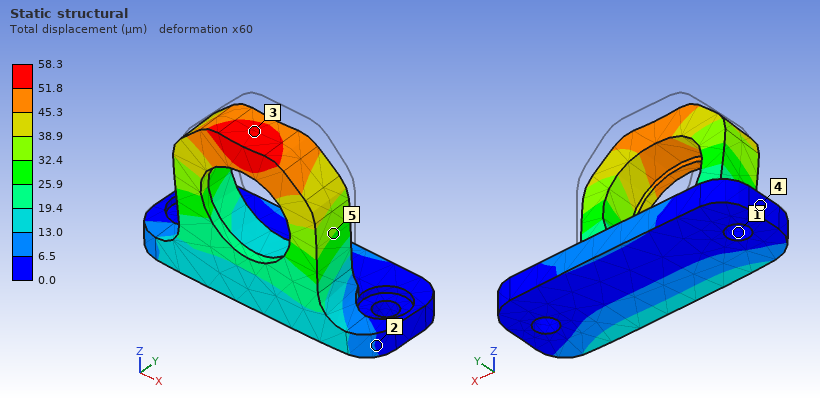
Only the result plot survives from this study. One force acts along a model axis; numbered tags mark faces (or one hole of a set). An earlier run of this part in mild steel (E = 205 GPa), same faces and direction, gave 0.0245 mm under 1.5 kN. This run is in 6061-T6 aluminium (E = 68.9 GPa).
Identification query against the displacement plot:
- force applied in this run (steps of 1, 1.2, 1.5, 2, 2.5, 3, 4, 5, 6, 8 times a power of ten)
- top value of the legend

1.2 kN
58.3 µm
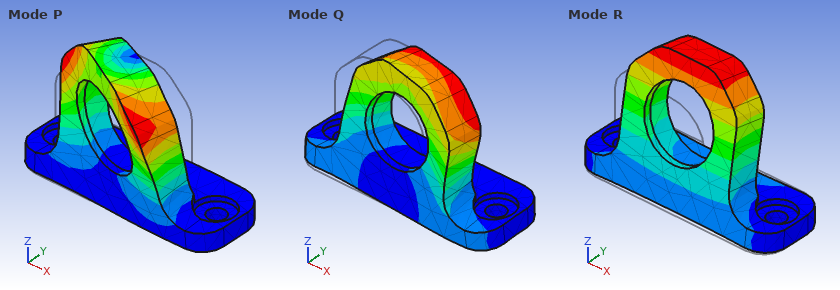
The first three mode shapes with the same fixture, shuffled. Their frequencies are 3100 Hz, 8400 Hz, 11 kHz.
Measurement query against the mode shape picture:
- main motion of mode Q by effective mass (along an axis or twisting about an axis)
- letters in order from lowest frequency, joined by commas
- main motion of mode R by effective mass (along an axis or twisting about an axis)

along X
R, Q, P
along Y
